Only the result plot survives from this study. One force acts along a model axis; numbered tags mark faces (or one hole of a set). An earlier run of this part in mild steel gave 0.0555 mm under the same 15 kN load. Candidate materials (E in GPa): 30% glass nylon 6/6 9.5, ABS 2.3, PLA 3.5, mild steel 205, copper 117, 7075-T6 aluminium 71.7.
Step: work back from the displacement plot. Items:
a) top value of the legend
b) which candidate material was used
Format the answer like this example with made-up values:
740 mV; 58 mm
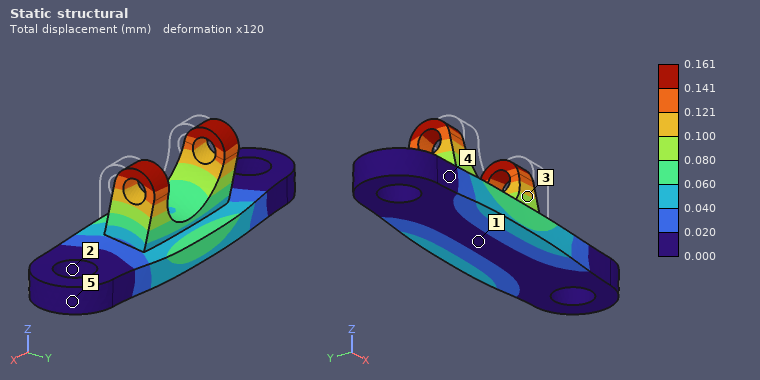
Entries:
0.161 mm; 7075-T6 aluminium
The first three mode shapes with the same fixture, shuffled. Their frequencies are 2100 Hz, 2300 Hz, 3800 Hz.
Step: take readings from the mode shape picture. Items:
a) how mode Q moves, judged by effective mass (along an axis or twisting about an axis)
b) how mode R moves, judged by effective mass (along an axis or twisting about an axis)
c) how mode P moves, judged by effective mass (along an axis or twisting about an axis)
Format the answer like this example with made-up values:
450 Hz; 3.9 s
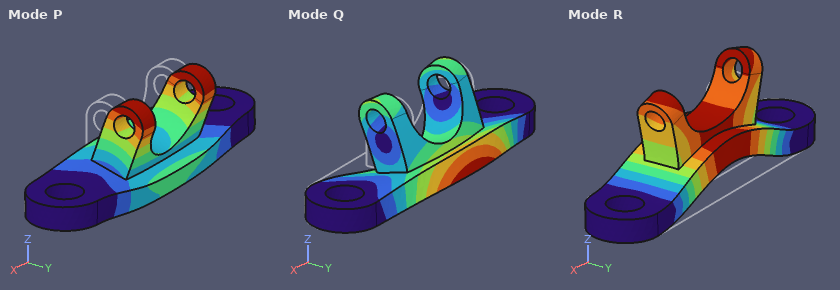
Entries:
along Y; along Z; along Y
